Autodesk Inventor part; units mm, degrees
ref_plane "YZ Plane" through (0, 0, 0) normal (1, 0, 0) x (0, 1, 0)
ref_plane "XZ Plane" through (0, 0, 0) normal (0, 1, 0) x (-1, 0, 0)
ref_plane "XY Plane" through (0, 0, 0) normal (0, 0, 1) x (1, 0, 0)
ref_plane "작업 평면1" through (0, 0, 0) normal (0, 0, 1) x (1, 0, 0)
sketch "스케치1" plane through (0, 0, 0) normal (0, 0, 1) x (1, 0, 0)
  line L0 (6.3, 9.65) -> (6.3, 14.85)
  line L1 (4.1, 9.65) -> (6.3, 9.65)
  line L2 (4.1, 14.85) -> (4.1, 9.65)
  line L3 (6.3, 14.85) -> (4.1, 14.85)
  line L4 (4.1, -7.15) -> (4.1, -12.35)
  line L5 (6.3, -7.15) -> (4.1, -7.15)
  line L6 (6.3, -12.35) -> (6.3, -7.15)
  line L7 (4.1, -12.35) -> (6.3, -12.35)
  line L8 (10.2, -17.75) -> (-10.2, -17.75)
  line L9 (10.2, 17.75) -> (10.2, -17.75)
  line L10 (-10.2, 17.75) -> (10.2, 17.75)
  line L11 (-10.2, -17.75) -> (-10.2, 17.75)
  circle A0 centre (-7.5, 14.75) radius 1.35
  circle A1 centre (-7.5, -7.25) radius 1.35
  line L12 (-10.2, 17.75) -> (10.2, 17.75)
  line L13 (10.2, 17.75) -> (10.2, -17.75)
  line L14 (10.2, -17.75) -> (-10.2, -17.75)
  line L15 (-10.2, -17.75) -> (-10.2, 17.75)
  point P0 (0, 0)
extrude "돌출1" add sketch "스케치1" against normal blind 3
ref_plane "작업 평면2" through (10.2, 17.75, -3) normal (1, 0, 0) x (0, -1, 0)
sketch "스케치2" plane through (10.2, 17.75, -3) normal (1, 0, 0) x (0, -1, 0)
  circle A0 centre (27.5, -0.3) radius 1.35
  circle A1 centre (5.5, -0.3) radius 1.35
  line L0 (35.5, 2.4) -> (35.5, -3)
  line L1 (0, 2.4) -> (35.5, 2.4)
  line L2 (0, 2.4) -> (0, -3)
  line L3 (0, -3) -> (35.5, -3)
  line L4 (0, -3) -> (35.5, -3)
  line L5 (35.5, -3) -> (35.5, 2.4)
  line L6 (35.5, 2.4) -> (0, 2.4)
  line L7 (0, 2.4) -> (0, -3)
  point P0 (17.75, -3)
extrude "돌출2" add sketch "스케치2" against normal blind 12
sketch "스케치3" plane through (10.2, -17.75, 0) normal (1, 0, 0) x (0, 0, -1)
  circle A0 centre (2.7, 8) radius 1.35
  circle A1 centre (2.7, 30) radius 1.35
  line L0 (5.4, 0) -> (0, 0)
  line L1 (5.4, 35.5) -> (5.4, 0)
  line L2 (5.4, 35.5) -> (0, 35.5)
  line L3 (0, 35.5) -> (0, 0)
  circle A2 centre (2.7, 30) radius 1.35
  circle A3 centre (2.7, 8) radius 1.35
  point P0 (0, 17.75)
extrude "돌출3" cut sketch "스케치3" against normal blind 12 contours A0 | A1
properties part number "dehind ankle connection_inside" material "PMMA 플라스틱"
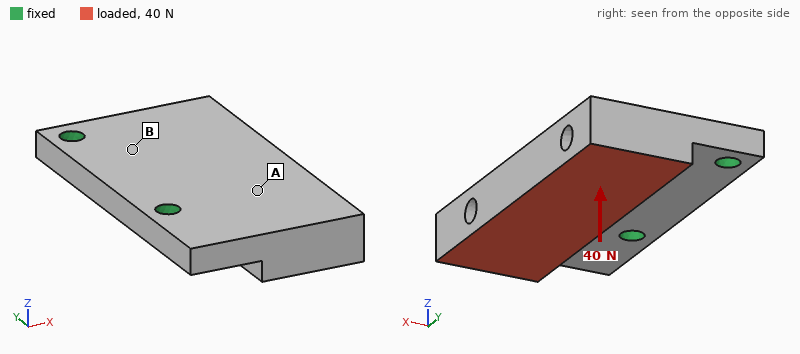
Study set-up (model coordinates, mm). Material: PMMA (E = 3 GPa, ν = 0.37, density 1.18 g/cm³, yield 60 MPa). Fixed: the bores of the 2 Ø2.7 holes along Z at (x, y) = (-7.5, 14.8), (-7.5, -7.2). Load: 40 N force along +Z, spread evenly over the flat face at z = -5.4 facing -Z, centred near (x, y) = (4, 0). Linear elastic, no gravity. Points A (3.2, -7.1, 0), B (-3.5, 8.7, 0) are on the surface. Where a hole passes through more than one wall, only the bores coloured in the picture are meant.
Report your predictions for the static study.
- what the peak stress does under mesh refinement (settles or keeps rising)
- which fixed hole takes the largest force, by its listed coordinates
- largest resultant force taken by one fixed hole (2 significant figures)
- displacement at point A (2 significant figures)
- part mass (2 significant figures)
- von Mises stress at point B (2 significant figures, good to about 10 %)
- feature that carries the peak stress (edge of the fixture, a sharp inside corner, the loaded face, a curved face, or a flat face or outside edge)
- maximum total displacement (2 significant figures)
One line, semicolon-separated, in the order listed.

keeps rising; (-7.5, -7.2); 26 N; 0.11 mm; 3.6 g; 4.3 MPa; edge of the fixture; 0.22 mm
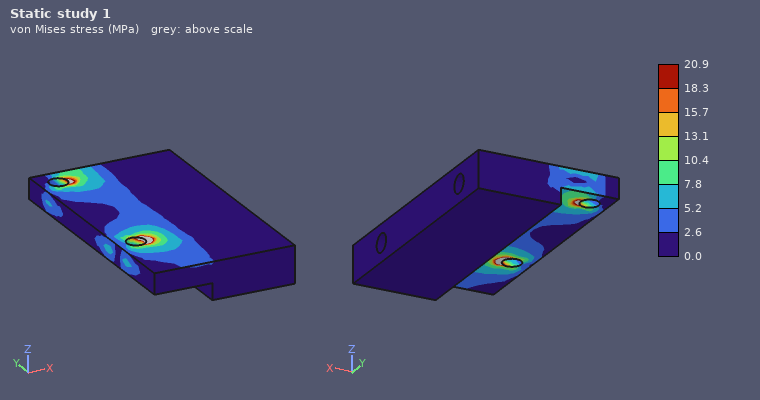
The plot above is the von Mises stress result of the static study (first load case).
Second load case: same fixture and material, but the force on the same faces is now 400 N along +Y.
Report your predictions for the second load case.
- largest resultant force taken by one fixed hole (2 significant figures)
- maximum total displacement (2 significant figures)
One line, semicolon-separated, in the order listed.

290 N; 0.26 mm
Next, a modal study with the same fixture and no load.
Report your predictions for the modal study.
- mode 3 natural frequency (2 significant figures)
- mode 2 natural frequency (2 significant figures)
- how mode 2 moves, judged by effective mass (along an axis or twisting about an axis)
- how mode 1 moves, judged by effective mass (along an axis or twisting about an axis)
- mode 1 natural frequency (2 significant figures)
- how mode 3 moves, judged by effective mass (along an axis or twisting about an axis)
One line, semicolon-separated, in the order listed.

6900 Hz; 3500 Hz; twisting about X; along Z; 1600 Hz; along Y
